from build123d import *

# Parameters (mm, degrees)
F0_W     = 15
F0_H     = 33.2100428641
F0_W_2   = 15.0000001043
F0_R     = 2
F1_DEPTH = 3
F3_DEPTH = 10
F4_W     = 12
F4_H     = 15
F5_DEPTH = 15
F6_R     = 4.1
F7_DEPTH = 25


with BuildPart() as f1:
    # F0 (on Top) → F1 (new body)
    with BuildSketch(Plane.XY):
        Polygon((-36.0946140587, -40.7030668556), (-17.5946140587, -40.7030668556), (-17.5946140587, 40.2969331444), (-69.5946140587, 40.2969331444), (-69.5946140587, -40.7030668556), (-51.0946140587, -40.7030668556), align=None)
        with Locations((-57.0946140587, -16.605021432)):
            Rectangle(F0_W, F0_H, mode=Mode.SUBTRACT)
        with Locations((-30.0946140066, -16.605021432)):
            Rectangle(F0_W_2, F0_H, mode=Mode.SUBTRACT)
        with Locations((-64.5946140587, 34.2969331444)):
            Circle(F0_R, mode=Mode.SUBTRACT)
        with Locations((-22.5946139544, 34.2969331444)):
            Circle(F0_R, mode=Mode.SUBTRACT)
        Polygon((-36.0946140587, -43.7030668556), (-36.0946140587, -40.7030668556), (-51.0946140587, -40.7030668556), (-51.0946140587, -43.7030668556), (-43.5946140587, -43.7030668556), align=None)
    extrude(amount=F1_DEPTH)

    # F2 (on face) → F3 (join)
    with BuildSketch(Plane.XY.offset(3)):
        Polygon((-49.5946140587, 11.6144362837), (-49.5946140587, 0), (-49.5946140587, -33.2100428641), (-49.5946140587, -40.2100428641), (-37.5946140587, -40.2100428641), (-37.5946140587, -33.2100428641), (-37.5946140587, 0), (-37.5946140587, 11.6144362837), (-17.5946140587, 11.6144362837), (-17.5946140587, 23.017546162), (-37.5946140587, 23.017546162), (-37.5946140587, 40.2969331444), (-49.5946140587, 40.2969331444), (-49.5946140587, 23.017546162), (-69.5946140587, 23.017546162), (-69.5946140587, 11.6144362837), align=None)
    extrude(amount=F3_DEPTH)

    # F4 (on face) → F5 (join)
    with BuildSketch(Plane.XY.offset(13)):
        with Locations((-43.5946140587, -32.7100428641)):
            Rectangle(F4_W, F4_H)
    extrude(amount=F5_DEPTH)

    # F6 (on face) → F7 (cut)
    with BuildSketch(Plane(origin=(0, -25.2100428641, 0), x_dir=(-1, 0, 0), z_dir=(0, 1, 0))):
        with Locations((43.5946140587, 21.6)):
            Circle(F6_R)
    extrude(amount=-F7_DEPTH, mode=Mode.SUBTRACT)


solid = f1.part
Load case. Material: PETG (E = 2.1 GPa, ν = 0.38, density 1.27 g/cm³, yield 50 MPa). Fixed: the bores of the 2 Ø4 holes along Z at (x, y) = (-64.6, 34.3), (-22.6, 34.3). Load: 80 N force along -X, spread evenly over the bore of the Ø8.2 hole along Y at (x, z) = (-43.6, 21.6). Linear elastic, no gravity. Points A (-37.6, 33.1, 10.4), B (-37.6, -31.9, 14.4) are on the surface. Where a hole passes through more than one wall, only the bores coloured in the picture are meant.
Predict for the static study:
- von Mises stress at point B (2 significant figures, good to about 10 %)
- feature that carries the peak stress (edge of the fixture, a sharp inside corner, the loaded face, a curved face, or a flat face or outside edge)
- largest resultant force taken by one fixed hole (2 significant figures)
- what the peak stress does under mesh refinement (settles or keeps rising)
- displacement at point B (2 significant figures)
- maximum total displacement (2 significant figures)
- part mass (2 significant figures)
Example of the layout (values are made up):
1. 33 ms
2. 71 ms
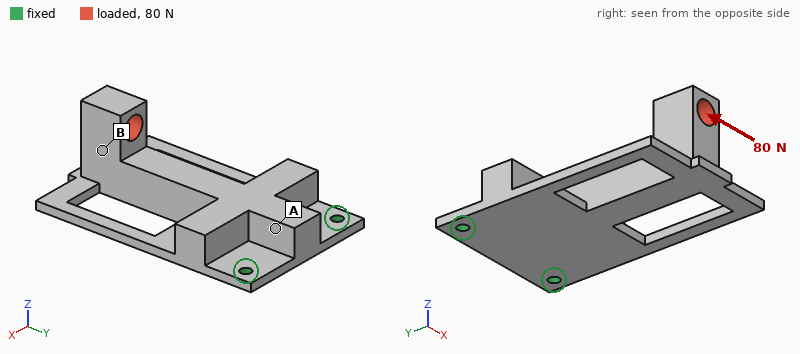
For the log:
1. 2.4 MPa
2. edge of the fixture
3. 140 N
4. keeps rising
5. 0.66 mm
6. 1.1 mm
7. 33 g
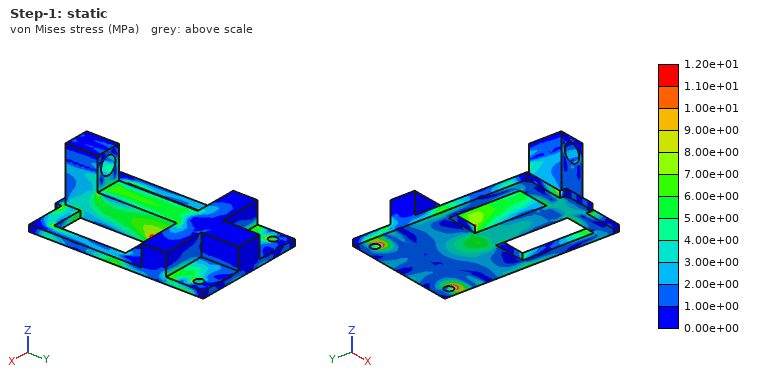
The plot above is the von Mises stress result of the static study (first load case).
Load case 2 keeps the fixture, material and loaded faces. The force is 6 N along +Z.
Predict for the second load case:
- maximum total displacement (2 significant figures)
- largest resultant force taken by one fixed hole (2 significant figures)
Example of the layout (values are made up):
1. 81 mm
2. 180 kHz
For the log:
1. 1.1 mm
2. 3.6 N
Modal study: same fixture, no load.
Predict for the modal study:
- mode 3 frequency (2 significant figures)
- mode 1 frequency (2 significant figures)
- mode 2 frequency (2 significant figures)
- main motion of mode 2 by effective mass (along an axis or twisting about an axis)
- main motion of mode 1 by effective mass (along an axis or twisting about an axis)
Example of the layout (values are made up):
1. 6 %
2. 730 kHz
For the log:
1. 850 Hz
2. 120 Hz
3. 680 Hz
4. along X
5. along Z
